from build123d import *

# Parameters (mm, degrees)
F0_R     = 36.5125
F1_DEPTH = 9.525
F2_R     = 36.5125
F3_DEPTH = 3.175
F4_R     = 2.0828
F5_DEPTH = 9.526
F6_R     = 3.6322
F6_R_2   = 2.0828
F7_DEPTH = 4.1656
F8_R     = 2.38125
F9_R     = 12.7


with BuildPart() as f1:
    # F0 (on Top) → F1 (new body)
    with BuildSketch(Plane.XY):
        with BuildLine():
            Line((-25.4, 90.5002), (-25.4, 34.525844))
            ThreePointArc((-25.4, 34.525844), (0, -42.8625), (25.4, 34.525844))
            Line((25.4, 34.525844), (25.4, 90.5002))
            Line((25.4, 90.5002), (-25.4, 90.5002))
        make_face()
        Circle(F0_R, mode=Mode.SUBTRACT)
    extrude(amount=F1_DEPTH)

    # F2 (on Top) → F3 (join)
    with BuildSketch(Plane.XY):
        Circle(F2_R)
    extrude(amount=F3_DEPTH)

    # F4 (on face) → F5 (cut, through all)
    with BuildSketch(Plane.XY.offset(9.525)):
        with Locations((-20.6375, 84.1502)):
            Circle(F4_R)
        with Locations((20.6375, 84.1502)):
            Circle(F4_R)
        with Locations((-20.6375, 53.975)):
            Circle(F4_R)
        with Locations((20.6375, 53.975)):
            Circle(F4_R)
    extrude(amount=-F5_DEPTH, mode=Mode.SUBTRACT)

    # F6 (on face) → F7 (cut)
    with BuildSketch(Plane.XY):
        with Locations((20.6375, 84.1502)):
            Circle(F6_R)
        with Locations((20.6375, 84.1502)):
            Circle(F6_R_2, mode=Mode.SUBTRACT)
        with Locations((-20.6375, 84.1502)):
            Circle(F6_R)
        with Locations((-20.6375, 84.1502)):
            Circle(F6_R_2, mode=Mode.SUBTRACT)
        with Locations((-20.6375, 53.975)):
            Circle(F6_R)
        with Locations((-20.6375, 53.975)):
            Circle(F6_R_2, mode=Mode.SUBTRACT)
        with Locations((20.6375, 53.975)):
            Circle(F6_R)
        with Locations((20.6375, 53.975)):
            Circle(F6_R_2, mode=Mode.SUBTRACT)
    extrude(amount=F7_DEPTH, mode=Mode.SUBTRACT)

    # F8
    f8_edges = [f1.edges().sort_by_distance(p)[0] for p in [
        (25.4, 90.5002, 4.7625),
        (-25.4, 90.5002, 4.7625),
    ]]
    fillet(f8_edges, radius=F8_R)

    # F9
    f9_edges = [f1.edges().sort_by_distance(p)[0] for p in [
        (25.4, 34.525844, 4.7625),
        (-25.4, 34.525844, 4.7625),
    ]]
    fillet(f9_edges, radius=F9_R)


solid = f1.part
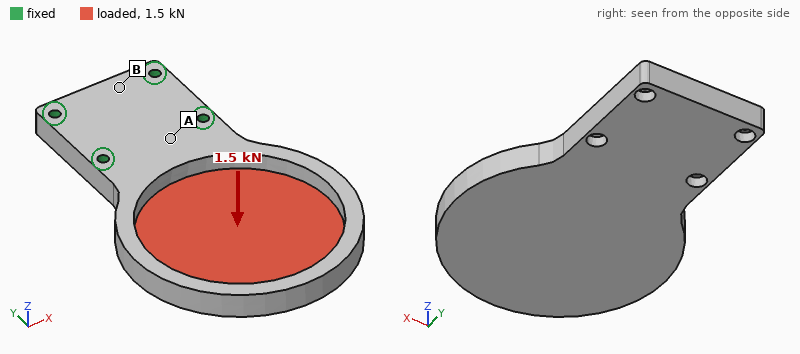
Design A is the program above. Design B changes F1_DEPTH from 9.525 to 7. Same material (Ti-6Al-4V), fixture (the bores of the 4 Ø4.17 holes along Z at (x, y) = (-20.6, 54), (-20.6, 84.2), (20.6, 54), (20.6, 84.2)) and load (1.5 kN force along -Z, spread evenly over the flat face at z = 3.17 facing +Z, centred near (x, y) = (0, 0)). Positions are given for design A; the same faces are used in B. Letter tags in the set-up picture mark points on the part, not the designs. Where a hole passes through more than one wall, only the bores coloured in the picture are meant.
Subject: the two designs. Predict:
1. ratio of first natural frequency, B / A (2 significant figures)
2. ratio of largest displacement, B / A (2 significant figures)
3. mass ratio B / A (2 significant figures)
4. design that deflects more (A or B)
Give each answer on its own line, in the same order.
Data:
0.76
2.1
0.80
B
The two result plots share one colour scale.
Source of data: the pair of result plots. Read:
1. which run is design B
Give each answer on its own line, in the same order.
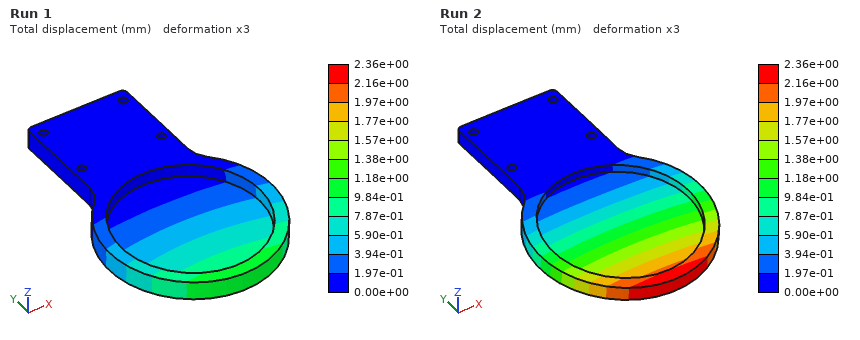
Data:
Run 2
